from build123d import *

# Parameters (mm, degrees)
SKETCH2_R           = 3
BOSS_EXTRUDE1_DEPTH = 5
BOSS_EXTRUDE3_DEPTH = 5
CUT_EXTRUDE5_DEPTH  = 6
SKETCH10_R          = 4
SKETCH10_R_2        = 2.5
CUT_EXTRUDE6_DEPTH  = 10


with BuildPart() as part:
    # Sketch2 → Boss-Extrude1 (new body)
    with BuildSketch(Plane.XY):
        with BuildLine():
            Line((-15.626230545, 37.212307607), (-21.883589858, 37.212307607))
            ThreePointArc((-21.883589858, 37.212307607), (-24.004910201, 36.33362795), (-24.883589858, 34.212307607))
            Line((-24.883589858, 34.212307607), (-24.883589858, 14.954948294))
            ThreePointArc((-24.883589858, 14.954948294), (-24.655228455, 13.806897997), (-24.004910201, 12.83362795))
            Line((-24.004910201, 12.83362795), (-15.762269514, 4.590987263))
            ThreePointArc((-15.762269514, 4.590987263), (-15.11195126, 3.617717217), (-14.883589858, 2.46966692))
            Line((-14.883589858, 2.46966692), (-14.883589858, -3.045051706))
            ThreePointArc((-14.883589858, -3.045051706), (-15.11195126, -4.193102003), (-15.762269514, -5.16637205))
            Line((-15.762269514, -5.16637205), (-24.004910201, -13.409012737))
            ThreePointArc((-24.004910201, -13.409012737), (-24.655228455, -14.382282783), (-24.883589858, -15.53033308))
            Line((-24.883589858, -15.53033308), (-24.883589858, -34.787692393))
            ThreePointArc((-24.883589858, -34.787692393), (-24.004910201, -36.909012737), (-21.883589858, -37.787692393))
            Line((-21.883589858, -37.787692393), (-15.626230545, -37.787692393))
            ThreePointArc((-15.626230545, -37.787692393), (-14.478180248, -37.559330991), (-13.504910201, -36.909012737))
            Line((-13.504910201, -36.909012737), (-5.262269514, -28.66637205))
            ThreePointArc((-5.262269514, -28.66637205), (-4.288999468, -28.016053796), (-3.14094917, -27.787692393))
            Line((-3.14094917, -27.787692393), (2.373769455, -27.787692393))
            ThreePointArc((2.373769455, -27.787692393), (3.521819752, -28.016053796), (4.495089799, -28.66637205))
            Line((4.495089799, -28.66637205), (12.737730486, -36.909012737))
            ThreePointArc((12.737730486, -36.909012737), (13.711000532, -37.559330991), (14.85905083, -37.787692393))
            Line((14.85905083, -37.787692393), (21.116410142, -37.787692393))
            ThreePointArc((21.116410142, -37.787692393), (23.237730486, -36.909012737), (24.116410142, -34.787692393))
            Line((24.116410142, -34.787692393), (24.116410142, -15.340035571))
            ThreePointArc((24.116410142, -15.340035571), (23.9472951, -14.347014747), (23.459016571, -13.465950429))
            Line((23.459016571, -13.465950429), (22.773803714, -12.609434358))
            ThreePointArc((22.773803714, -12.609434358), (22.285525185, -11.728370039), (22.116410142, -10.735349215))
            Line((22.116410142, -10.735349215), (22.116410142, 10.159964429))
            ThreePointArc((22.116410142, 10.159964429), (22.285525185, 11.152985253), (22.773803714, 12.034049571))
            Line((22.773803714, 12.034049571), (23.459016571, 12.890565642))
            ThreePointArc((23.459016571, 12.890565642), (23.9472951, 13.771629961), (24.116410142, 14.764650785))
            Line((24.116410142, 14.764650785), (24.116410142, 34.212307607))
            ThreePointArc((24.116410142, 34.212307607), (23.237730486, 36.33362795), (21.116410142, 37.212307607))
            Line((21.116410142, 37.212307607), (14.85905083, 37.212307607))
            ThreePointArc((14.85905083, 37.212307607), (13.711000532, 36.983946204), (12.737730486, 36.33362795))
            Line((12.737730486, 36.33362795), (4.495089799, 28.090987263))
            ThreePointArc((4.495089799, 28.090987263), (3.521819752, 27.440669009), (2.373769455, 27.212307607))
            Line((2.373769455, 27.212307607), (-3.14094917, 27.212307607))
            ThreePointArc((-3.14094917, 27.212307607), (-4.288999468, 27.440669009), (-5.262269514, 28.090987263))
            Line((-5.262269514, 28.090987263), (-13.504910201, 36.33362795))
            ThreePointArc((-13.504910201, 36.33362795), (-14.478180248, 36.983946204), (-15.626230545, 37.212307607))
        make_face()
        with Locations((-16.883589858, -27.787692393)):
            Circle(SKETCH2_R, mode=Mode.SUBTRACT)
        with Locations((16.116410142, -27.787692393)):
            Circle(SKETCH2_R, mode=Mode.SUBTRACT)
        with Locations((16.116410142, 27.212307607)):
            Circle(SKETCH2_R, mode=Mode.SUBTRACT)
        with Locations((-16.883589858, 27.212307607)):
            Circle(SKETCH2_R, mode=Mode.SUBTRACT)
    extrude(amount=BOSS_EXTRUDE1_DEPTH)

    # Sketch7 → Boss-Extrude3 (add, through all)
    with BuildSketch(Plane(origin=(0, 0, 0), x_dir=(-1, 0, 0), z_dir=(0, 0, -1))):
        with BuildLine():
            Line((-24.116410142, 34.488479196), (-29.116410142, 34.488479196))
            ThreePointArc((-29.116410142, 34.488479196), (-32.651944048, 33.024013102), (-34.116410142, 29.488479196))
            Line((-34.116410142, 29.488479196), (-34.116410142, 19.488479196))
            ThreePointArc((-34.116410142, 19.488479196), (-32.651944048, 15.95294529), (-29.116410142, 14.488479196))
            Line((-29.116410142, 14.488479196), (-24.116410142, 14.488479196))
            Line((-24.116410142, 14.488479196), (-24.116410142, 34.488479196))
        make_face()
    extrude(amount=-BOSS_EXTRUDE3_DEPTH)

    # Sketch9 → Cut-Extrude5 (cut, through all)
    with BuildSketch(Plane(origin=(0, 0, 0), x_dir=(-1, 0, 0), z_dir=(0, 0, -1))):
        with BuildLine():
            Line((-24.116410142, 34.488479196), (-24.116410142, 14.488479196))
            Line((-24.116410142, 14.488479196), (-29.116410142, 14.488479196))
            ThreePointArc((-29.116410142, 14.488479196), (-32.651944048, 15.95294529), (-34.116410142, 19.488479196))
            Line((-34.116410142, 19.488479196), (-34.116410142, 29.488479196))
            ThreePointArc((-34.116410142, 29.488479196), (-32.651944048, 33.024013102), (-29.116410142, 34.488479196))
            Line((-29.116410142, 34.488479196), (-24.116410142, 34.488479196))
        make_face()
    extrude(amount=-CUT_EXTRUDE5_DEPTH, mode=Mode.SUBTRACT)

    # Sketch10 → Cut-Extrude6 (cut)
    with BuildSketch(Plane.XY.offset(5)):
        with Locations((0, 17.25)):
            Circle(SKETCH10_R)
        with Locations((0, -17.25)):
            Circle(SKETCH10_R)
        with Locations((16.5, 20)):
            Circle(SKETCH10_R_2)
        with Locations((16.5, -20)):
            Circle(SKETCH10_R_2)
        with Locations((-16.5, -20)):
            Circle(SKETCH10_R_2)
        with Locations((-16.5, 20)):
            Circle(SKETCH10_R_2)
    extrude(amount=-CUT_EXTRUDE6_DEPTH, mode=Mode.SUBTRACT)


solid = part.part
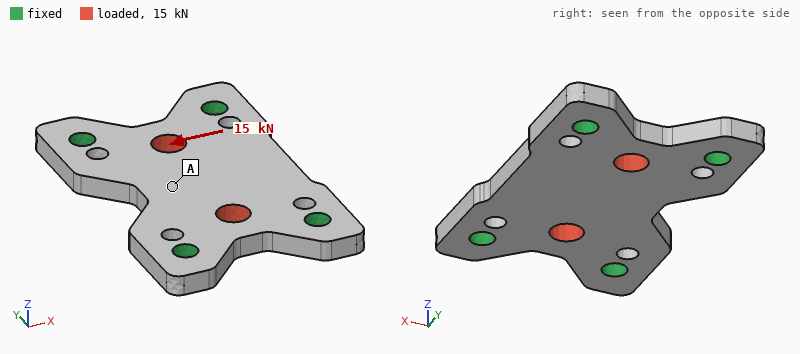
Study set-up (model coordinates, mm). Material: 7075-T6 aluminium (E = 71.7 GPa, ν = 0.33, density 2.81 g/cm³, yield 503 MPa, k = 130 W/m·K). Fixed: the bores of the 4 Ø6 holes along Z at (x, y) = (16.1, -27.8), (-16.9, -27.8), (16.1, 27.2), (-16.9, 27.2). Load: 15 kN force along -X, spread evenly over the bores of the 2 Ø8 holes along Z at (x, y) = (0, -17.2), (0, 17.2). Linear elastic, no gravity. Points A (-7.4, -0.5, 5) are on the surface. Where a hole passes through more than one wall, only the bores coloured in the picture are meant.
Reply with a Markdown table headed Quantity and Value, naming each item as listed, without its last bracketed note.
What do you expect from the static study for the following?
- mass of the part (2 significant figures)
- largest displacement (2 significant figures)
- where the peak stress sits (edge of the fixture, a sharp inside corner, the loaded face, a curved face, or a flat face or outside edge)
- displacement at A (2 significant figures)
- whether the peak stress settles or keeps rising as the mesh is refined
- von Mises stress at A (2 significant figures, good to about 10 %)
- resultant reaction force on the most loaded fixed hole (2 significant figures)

| Quantity | Value |
|---|---|
| mass of the part | 39 g |
| largest displacement | 28 µm |
| where the peak stress sits | edge of the fixture |
| displacement at A | 23 µm |
| whether the peak stress settles or keeps rising as the mesh is refined | keeps rising |
| von Mises stress at A | 16 MPa |
| resultant reaction force on the most loaded fixed hole | 4.3 kN |
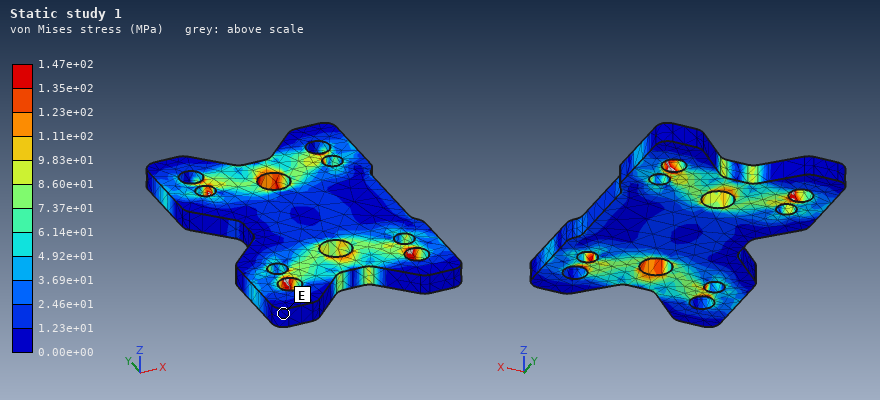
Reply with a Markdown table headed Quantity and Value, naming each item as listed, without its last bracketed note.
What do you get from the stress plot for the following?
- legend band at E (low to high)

| Quantity | Value |
|---|---|
| legend band at E | 0.00e+00 to 1.23e+01 MPa |
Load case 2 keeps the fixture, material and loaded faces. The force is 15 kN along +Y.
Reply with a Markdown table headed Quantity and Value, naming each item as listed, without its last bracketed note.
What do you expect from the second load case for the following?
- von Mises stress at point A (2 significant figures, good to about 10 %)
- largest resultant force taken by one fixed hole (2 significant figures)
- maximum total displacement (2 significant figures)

| Quantity | Value |
|---|---|
| von Mises stress at point A | 32 MPa |
| largest resultant force taken by one fixed hole | 4.4 kN |
| maximum total displacement | 25 µm |
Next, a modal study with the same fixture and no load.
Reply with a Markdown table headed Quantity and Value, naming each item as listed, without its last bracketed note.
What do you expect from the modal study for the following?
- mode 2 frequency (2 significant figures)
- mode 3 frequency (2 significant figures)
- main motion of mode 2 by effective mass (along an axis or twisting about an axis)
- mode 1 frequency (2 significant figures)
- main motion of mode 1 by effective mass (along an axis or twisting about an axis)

| Quantity | Value |
|---|---|
| mode 2 frequency | 12 kHz |
| mode 3 frequency | 19 kHz |
| main motion of mode 2 by effective mass | twisting about Y |
| mode 1 frequency | 7900 Hz |
| main motion of mode 1 by effective mass | along Z |
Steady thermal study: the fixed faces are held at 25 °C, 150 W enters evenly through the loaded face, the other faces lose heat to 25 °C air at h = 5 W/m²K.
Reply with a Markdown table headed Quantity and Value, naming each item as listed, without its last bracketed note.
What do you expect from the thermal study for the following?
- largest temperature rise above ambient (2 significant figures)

| Quantity | Value |
|---|---|
| largest temperature rise above ambient | 61 K |
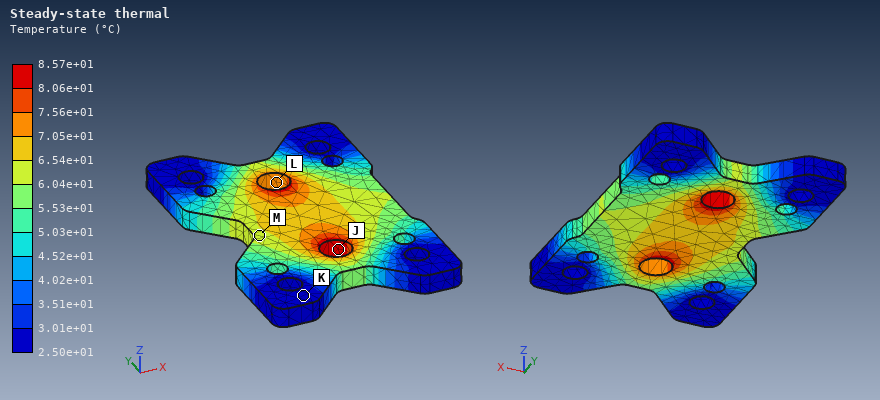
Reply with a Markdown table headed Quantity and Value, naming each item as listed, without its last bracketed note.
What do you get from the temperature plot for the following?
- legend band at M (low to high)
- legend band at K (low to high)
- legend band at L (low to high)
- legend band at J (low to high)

| Quantity | Value |
|---|---|
| legend band at M | 6.04e+01 to 6.54e+01 °C |
| legend band at K | 2.50e+01 to 3.01e+01 °C |
| legend band at L | 7.05e+01 to 7.56e+01 °C |
| legend band at J | 8.06e+01 to 8.57e+01 °C |
